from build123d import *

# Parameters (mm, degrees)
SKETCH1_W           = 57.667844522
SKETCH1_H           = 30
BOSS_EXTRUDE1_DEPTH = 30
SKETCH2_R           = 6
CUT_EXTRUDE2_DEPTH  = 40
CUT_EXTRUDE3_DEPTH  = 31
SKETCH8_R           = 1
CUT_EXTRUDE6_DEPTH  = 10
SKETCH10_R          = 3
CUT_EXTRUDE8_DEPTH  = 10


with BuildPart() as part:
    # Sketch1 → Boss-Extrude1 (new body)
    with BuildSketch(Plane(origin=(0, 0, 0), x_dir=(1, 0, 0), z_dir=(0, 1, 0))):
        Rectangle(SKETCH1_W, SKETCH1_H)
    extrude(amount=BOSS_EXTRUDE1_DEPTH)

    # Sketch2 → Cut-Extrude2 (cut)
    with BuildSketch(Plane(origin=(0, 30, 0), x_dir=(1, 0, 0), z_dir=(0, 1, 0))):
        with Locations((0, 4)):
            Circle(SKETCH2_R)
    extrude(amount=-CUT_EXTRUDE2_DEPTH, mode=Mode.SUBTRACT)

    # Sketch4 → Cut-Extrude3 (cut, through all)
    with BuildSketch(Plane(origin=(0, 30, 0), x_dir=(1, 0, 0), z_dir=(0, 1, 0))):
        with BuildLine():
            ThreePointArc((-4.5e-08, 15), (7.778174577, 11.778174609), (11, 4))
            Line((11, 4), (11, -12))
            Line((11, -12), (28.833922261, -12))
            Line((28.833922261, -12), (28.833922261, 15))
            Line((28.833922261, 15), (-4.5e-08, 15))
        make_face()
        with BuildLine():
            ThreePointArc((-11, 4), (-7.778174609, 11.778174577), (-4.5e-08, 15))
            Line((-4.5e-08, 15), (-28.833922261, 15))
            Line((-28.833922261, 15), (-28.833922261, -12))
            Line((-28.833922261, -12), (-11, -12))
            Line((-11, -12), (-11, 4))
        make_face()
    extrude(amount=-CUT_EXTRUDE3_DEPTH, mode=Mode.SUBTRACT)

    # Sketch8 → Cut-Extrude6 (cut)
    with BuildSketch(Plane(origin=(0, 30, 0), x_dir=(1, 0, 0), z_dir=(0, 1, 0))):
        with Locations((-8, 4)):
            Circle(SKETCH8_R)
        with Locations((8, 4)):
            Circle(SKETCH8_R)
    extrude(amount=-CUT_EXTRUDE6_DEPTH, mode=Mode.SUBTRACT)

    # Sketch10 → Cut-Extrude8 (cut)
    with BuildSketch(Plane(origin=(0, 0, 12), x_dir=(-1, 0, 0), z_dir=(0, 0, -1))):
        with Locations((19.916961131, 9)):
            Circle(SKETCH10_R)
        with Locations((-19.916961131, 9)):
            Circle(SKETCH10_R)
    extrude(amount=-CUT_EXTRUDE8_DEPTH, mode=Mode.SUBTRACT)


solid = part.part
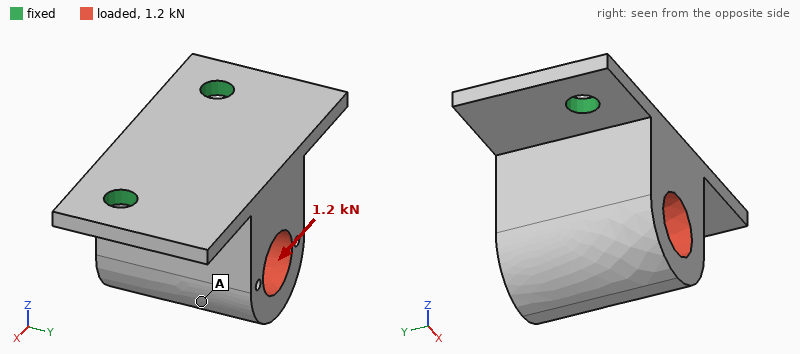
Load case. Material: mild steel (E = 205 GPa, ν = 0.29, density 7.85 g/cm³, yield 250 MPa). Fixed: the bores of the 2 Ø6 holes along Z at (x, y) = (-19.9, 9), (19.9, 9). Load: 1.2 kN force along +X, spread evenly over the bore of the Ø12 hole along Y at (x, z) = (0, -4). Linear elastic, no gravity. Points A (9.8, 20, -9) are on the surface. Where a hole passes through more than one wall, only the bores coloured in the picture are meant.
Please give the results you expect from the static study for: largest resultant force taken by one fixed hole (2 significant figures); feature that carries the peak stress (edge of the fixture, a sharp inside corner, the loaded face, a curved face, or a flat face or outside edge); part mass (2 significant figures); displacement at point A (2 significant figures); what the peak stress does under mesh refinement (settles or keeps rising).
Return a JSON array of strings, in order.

["940 N", "edge of the fixture", "140 g", "13 µm", "keeps rising"]
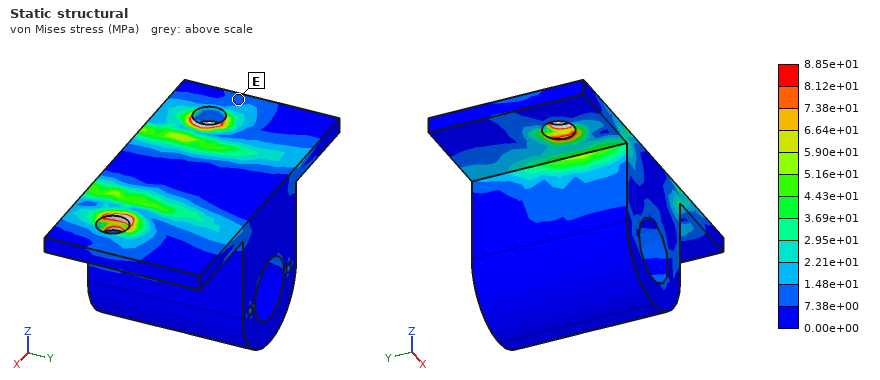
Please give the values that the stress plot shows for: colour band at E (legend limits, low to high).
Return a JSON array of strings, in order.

["7.38e+00 to 1.48e+01 MPa"]
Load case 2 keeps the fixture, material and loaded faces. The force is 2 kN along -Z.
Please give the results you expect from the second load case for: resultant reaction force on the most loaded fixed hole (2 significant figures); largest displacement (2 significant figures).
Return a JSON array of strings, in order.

["1.1 kN", "64 µm"]
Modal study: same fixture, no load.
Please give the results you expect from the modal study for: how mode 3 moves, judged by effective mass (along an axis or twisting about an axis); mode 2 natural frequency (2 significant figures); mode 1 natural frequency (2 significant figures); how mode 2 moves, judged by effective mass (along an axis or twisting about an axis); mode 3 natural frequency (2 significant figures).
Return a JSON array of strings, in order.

["along Z", "6100 Hz", "2100 Hz", "along X", "7000 Hz"]
